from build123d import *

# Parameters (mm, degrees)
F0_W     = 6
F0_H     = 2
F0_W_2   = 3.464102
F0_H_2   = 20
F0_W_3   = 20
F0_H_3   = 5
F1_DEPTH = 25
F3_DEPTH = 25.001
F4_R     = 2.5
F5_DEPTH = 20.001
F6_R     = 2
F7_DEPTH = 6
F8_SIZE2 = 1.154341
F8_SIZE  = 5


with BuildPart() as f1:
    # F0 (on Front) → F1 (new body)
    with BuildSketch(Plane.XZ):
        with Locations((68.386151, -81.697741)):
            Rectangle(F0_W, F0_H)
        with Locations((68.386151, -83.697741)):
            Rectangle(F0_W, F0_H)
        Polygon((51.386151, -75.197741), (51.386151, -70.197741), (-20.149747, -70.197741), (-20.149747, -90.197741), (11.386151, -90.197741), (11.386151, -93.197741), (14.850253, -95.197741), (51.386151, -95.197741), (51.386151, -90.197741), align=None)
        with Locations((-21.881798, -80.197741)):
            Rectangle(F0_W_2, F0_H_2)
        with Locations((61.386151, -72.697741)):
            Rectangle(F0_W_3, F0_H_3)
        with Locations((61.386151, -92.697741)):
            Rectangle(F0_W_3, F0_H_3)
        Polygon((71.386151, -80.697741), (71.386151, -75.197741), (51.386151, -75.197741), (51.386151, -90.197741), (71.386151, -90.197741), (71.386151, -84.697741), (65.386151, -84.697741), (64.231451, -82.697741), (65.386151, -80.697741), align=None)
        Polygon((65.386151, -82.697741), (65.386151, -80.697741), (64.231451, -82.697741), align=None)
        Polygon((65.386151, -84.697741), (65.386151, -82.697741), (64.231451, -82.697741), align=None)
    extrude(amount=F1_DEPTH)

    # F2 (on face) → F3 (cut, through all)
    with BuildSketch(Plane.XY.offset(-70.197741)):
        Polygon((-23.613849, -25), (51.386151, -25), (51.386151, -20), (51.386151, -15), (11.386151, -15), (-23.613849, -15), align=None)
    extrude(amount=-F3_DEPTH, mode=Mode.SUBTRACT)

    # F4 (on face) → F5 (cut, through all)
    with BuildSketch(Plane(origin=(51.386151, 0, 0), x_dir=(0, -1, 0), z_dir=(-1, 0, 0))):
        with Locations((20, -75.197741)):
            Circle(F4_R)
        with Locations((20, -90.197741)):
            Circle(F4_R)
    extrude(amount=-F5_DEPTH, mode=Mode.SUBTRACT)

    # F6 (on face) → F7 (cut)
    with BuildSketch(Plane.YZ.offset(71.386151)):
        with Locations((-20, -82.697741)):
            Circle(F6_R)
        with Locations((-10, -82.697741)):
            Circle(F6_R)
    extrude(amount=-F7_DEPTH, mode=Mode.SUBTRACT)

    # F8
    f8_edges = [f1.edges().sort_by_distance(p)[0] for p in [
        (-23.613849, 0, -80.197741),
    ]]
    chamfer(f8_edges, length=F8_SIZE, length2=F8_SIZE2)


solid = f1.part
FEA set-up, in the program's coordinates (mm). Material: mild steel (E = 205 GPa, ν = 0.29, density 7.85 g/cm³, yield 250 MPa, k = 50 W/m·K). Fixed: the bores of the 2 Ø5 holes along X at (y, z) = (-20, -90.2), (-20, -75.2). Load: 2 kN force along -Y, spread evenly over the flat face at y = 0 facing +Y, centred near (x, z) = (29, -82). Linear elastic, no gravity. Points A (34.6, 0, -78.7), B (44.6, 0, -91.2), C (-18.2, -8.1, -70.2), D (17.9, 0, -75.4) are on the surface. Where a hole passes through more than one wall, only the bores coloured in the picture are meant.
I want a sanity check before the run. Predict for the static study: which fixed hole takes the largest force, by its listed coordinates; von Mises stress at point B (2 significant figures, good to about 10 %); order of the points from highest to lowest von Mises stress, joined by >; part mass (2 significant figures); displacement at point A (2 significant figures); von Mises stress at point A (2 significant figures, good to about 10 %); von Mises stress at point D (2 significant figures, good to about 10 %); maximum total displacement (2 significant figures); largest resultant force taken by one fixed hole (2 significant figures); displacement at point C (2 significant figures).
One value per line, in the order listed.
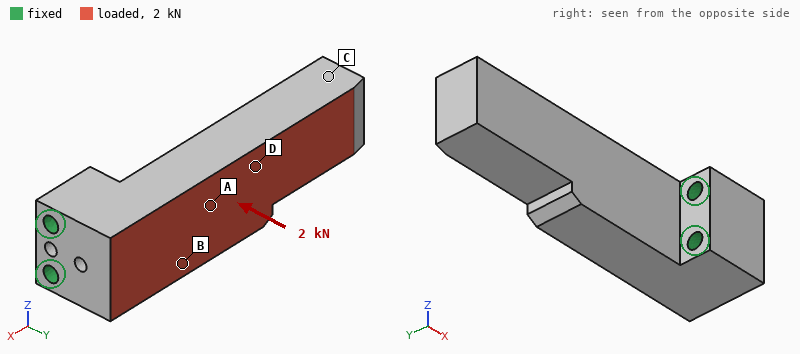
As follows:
(-20, -75.2)
45 MPa
B > A > D > C
290 g
17 µm
31 MPa
15 MPa
83 µm
1.2 kN
76 µm
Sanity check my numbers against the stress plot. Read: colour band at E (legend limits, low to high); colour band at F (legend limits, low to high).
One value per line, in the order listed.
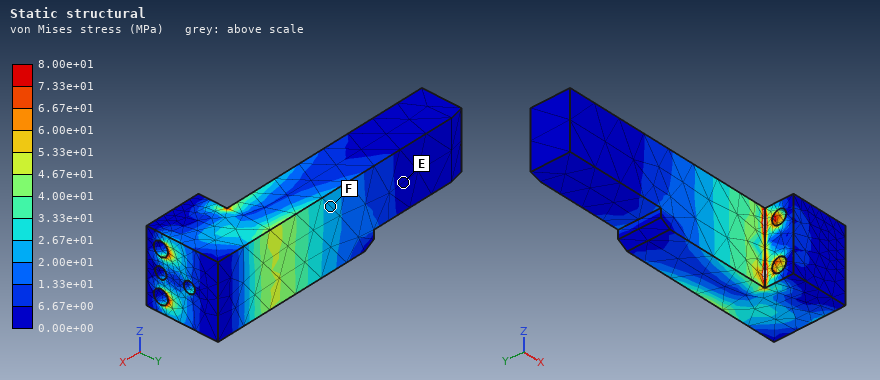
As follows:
0.00e+00 to 6.67e+00 MPa
2.00e+01 to 2.67e+01 MPa
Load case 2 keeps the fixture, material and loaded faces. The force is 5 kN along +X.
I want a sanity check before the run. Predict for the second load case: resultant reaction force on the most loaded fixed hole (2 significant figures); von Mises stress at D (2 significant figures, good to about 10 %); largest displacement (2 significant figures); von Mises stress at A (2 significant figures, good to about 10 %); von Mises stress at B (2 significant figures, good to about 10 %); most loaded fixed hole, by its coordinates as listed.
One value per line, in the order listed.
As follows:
2.6 kN
22 MPa
72 µm
31 MPa
37 MPa
(-20, -75.2)
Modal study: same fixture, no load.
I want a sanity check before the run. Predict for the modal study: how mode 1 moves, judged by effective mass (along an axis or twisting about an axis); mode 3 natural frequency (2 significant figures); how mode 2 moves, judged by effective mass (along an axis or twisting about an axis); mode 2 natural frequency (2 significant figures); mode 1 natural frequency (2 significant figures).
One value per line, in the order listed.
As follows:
along Y
9100 Hz
along Z
2600 Hz
1800 Hz
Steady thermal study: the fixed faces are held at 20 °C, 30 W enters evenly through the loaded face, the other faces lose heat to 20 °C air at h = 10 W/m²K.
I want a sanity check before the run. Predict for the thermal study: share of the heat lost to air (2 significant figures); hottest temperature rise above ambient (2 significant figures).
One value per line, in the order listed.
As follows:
6.5 %
55 K
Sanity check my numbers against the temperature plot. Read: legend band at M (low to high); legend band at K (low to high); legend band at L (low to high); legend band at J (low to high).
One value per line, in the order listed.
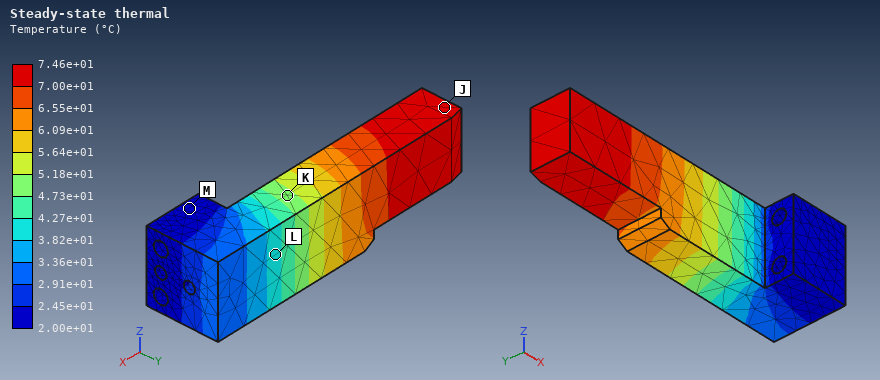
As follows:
2.00e+01 to 2.45e+01 °C
4.73e+01 to 5.18e+01 °C
3.82e+01 to 4.27e+01 °C
7.00e+01 to 7.46e+01 °C
